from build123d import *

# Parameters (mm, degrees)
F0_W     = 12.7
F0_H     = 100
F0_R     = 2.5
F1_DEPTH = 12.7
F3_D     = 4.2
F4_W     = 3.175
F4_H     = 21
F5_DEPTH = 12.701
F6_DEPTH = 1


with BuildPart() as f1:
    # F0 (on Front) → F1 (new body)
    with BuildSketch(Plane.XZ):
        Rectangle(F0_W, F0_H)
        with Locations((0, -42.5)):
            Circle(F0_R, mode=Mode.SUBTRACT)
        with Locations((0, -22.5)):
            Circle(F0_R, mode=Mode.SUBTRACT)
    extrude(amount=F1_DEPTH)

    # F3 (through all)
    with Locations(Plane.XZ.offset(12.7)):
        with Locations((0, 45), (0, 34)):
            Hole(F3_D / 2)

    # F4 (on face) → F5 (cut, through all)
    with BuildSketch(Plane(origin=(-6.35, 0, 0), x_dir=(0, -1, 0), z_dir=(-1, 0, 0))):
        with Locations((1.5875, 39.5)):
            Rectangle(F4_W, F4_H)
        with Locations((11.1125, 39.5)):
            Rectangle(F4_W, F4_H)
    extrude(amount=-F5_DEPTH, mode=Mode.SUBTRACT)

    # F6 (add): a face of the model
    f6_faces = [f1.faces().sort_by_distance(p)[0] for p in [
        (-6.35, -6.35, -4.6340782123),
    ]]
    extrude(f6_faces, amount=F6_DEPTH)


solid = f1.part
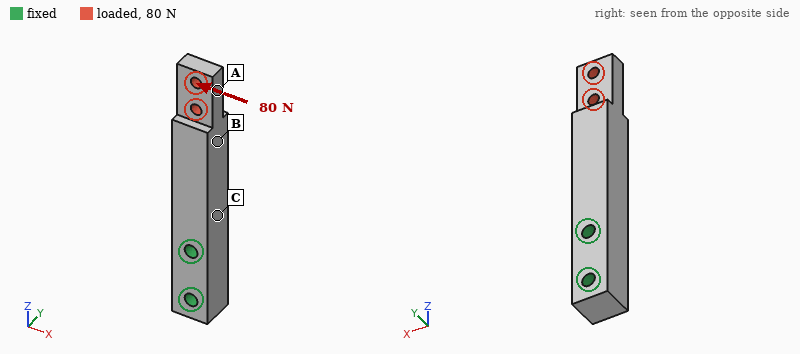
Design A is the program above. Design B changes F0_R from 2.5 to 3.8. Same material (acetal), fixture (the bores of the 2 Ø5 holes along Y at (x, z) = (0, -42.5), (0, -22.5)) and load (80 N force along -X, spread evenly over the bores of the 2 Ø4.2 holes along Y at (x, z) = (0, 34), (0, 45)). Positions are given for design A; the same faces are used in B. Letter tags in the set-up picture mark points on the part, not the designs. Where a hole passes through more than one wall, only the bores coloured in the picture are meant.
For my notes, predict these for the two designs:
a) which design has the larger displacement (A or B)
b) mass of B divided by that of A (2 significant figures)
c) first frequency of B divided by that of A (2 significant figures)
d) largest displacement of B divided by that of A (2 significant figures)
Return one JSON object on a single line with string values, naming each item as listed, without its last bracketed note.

{"which design has the larger displacement": "A", "mass of B divided by that of A": "0.96", "first frequency of B divided by that of A": "1.1", "largest displacement of B divided by that of A": "0.89"}
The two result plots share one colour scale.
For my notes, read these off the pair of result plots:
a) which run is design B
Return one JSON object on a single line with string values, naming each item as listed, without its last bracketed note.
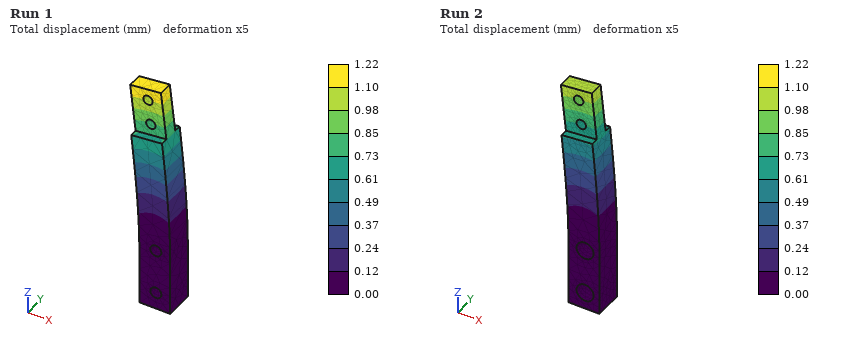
{"which run is design B": "Run 2"}
